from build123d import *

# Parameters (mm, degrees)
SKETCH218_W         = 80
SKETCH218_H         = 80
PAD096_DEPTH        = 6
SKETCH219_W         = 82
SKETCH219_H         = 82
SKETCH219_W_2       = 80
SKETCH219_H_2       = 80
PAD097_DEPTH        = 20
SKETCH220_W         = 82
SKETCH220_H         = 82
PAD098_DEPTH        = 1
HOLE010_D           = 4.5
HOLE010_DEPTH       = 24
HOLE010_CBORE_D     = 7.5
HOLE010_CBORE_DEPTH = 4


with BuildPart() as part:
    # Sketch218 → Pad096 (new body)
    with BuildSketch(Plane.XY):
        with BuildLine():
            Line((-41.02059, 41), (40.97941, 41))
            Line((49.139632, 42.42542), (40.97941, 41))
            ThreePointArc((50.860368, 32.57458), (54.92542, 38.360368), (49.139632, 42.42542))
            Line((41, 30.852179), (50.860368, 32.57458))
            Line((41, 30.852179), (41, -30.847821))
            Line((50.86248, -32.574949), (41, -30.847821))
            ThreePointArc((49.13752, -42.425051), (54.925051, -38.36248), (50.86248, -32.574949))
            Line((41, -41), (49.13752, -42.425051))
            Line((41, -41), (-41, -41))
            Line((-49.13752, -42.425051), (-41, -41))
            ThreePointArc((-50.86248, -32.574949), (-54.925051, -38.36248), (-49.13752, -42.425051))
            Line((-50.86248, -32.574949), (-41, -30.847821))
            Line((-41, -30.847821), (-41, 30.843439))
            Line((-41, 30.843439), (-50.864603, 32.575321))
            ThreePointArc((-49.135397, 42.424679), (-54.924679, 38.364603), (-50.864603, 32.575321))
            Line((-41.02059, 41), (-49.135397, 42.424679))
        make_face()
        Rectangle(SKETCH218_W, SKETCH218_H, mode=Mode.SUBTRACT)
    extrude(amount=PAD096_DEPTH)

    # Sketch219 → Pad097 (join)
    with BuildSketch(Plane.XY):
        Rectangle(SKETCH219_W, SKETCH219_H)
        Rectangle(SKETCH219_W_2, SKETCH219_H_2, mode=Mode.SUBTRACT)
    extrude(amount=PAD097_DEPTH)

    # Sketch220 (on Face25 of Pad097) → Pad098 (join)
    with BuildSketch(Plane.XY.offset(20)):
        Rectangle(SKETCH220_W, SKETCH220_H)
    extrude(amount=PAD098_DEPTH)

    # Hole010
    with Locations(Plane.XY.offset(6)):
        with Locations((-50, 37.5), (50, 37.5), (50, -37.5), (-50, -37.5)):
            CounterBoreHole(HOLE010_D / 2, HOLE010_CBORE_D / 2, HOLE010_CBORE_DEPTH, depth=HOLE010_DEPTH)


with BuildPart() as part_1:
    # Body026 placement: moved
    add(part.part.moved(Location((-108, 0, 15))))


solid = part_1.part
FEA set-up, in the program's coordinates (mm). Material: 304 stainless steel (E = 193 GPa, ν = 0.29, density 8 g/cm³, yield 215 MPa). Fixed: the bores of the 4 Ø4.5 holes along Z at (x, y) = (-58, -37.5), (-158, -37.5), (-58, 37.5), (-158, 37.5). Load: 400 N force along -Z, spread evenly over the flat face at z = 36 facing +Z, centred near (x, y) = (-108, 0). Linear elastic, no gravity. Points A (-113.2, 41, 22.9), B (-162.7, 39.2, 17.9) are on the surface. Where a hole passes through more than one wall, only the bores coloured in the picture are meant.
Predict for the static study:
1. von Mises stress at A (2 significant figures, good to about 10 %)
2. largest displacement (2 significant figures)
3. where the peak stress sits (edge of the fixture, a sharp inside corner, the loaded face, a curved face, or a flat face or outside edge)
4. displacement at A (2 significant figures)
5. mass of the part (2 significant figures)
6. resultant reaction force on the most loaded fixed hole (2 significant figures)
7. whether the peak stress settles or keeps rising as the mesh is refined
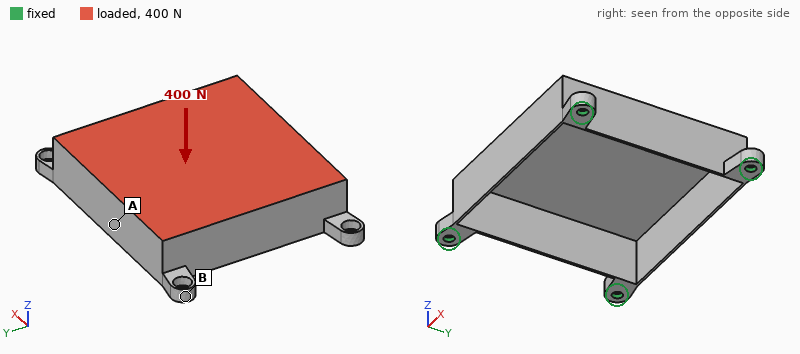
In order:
23 MPa
0.32 mm
a sharp inside corner
0.092 mm
120 g
140 N
keeps rising
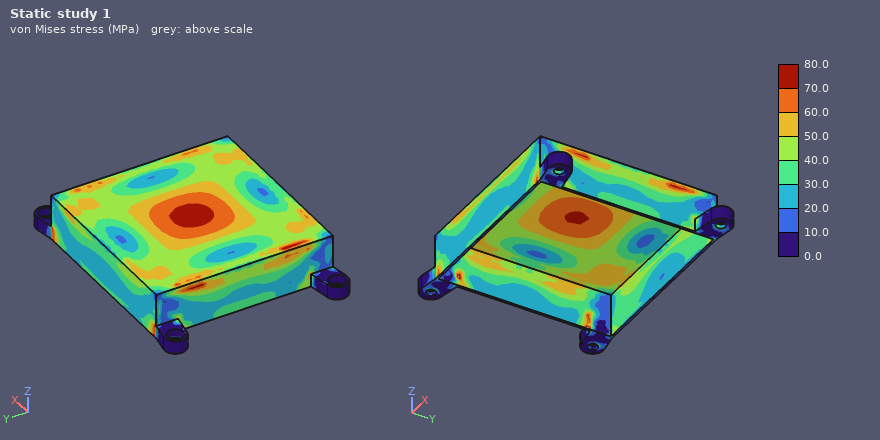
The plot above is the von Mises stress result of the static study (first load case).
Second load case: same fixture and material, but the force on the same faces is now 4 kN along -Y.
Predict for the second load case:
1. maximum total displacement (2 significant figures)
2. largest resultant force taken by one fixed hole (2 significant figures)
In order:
39 µm
1.1 kN
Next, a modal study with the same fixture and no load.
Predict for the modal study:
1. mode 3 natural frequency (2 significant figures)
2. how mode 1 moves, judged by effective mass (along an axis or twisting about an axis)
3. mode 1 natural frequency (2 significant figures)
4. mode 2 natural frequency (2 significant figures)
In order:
1900 Hz
along Z
930 Hz
1600 Hz
